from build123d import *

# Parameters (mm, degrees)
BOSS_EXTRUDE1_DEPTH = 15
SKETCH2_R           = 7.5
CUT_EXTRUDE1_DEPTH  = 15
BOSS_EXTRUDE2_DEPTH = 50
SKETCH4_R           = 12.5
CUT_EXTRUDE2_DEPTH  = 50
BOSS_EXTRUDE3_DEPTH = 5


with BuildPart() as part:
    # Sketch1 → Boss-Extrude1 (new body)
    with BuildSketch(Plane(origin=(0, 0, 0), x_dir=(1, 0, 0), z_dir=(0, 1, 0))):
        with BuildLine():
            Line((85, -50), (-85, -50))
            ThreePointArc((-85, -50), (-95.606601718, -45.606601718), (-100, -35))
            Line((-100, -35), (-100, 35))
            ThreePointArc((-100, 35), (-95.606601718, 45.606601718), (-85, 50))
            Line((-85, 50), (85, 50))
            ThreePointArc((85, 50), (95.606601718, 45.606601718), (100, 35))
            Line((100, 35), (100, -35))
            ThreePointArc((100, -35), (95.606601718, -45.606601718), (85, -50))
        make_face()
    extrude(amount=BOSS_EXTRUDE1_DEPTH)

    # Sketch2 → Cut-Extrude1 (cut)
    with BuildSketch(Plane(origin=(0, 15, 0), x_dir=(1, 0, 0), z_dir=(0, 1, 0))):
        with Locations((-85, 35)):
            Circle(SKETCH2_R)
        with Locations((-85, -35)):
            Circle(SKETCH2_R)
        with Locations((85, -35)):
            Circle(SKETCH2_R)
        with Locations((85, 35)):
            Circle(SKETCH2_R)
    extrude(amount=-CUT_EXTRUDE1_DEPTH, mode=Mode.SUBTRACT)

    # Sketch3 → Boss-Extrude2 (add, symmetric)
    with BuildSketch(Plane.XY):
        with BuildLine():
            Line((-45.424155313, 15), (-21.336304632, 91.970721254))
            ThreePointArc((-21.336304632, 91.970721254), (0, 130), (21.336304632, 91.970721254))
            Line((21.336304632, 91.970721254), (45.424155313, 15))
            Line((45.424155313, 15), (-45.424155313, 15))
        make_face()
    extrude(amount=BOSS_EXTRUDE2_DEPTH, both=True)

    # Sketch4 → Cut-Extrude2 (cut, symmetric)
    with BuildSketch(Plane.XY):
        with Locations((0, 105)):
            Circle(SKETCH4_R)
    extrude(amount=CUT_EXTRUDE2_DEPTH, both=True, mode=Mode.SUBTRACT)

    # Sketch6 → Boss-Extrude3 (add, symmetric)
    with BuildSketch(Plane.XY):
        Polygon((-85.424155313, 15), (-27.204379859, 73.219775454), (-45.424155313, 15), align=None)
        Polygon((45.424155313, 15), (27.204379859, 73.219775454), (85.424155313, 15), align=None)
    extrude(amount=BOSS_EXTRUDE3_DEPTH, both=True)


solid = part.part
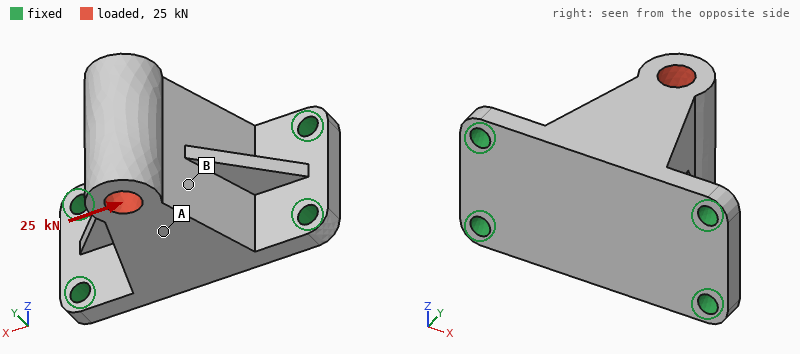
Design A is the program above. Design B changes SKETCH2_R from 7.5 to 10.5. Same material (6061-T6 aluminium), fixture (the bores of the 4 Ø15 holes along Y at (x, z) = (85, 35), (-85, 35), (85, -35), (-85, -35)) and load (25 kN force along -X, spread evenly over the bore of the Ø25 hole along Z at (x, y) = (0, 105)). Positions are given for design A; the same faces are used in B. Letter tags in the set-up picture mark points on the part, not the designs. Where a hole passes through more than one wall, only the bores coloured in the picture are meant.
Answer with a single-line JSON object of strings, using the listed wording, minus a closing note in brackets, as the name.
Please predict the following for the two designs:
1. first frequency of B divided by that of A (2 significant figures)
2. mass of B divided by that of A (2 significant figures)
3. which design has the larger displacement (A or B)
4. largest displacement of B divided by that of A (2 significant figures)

{"first frequency of B divided by that of A": "1.1", "mass of B divided by that of A": "0.99", "which design has the larger displacement": "A", "largest displacement of B divided by that of A": "0.92"}
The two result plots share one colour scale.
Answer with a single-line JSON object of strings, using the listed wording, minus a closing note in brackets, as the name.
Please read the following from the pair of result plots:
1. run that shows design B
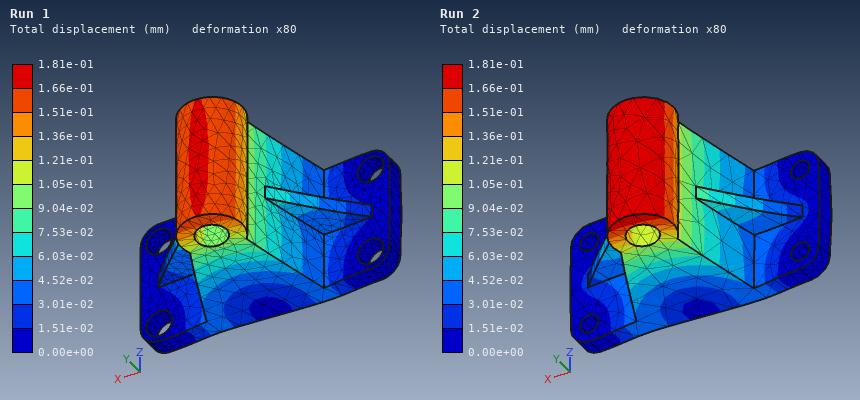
{"run that shows design B": "Run 1"}
